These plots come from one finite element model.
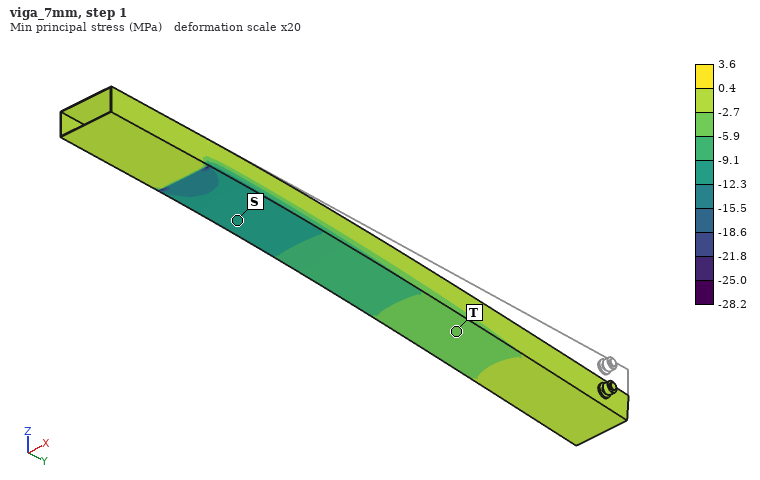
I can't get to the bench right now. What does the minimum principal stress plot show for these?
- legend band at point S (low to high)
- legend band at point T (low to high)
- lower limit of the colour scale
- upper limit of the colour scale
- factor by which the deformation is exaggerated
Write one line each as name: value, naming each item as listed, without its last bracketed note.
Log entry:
legend band at point S: -12.3 to -9.1 MPa
legend band at point T: -5.9 to -2.7 MPa
lower limit of the colour scale: -28.2 MPa
upper limit of the colour scale: 3.6 MPa
factor by which the deformation is exaggerated: 20
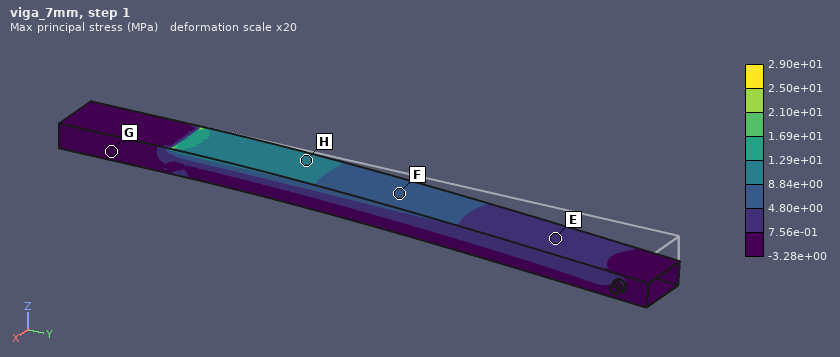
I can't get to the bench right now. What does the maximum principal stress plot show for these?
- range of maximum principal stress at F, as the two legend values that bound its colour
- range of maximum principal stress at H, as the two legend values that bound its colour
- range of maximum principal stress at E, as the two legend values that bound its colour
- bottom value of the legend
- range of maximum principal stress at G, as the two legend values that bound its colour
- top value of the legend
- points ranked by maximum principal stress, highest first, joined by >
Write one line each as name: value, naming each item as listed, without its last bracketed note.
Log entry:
range of maximum principal stress at F, as the two legend values that bound its colour: 4.80e+00 to 8.84e+00 MPa
range of maximum principal stress at H, as the two legend values that bound its colour: 8.84e+00 to 1.29e+01 MPa
range of maximum principal stress at E, as the two legend values that bound its colour: 7.56e-01 to 4.80e+00 MPa
bottom value of the legend: -3.28e+00 MPa
range of maximum principal stress at G, as the two legend values that bound its colour: -3.28e+00 to 7.56e-01 MPa
top value of the legend: 2.90e+01 MPa
points ranked by maximum principal stress, highest first, joined by >: H > F > E > G
